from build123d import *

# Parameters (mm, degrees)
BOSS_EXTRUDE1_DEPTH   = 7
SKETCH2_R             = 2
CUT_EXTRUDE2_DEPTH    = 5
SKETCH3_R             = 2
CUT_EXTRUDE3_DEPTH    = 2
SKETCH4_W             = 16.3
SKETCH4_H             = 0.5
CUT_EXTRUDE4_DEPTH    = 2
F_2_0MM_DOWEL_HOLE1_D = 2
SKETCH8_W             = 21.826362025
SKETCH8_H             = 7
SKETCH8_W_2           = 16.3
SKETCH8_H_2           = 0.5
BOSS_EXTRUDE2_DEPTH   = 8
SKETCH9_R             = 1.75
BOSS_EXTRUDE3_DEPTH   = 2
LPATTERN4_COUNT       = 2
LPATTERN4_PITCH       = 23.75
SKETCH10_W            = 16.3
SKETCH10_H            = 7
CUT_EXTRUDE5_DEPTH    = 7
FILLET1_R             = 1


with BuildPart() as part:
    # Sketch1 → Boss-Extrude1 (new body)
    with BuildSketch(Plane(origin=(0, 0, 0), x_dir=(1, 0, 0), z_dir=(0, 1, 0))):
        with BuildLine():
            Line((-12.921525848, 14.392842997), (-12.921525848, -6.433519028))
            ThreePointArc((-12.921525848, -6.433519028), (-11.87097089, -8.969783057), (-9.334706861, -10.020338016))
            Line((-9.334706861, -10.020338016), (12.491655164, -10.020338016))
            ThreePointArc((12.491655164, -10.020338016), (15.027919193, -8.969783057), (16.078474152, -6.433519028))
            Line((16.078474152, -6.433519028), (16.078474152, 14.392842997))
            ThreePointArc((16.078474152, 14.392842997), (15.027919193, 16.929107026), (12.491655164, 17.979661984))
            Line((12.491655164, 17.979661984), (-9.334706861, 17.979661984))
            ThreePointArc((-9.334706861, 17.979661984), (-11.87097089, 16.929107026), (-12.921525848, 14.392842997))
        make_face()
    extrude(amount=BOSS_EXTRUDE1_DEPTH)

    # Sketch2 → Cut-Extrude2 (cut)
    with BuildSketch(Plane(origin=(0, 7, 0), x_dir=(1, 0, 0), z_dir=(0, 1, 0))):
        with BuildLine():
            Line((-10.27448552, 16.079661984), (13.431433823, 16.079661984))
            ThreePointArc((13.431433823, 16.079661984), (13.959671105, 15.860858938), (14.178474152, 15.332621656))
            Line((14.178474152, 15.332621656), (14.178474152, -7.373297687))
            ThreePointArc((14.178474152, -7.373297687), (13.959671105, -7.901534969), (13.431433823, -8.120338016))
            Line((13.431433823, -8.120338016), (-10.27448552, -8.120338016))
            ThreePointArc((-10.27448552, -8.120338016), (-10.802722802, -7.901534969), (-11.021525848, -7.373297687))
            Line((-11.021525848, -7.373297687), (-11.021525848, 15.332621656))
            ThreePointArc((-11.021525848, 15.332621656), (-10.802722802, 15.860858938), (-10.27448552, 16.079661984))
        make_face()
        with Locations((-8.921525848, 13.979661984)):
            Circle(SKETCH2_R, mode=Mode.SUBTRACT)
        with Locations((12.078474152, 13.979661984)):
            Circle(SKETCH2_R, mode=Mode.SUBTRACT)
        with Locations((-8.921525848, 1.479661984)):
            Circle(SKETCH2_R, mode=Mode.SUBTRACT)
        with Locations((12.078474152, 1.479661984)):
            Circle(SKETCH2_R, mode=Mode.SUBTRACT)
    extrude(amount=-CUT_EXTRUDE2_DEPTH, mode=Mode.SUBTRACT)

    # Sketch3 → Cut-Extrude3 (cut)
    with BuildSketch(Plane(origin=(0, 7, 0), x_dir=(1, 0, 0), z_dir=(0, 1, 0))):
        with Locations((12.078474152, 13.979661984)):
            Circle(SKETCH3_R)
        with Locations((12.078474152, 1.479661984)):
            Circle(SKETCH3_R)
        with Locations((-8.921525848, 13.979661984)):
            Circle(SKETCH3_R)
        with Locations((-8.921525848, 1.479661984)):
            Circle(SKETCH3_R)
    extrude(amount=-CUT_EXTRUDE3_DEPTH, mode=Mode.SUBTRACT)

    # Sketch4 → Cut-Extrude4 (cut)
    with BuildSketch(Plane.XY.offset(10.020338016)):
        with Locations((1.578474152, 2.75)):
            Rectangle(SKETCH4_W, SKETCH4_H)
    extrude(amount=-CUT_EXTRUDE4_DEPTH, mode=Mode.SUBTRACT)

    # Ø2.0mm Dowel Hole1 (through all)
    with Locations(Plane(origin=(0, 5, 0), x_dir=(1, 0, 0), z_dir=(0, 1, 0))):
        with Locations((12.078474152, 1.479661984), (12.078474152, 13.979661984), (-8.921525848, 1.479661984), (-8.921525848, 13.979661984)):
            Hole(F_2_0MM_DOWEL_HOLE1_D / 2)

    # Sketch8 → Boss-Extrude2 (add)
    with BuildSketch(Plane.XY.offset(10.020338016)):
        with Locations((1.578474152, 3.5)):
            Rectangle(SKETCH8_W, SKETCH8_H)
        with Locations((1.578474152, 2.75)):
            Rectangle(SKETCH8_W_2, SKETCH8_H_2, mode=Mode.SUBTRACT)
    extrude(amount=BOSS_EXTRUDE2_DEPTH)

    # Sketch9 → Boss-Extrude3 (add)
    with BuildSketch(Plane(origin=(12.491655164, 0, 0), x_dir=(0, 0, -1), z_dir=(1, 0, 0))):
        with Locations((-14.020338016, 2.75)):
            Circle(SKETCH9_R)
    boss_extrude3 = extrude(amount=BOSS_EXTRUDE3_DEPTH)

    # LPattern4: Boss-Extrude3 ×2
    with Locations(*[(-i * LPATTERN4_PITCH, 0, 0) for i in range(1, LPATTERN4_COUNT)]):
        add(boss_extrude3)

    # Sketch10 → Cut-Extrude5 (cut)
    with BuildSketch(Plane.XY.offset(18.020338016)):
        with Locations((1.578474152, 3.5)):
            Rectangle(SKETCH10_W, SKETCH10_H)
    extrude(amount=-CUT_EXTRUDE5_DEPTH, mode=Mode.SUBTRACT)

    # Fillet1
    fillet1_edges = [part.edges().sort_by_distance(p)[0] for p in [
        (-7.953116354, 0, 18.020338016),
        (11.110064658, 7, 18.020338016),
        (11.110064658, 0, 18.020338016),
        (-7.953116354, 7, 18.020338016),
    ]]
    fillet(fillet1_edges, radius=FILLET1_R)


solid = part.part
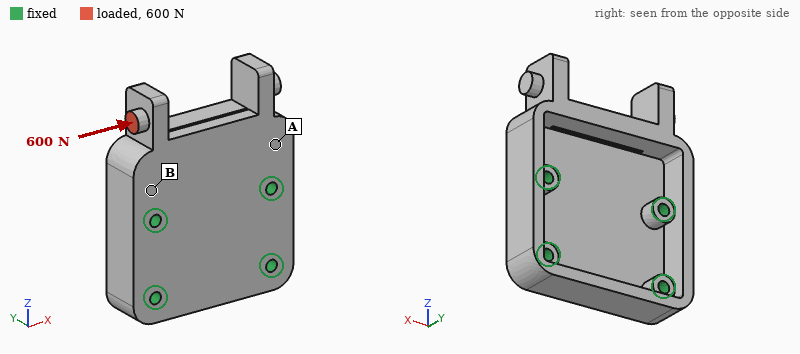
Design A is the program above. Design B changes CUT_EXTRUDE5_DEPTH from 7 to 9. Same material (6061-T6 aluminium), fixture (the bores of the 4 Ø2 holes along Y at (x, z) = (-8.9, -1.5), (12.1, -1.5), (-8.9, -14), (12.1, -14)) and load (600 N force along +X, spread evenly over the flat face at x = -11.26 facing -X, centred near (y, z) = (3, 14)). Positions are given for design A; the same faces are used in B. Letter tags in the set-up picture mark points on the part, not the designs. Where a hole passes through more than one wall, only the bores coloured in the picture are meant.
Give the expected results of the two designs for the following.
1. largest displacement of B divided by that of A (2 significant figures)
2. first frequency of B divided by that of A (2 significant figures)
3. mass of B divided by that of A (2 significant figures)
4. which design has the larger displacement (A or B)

2.2
1.1
0.93
B
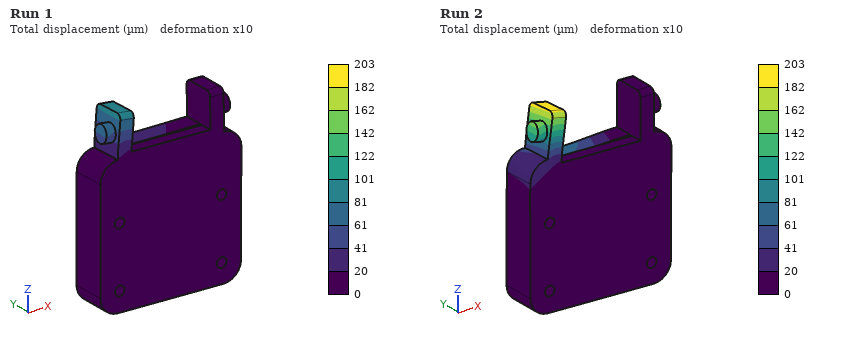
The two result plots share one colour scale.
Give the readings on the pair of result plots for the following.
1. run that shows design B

Run 2
